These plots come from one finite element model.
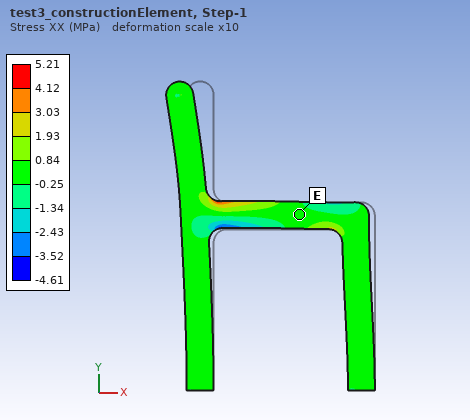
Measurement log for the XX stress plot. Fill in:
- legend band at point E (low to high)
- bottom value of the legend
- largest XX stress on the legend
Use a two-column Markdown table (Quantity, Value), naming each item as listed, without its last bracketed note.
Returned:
| Quantity | Value |
|---|---|
| legend band at point E | -0.25 to 0.84 MPa |
| bottom value of the legend | -4.61 MPa |
| largest XX stress on the legend | 5.21 MPa |
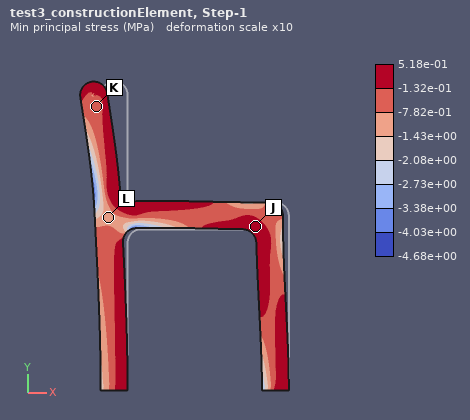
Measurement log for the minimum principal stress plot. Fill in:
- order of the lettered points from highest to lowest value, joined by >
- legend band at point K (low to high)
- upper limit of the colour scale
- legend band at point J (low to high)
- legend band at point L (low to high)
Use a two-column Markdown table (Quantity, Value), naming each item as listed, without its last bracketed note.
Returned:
| Quantity | Value |
|---|---|
| order of the lettered points from highest to lowest value, joined by > | J > K > L |
| legend band at point K | -7.82e-01 to -1.32e-01 MPa |
| upper limit of the colour scale | 5.18e-01 MPa |
| legend band at point J | -1.32e-01 to 5.18e-01 MPa |
| legend band at point L | -1.43e+00 to -7.82e-01 MPa |
